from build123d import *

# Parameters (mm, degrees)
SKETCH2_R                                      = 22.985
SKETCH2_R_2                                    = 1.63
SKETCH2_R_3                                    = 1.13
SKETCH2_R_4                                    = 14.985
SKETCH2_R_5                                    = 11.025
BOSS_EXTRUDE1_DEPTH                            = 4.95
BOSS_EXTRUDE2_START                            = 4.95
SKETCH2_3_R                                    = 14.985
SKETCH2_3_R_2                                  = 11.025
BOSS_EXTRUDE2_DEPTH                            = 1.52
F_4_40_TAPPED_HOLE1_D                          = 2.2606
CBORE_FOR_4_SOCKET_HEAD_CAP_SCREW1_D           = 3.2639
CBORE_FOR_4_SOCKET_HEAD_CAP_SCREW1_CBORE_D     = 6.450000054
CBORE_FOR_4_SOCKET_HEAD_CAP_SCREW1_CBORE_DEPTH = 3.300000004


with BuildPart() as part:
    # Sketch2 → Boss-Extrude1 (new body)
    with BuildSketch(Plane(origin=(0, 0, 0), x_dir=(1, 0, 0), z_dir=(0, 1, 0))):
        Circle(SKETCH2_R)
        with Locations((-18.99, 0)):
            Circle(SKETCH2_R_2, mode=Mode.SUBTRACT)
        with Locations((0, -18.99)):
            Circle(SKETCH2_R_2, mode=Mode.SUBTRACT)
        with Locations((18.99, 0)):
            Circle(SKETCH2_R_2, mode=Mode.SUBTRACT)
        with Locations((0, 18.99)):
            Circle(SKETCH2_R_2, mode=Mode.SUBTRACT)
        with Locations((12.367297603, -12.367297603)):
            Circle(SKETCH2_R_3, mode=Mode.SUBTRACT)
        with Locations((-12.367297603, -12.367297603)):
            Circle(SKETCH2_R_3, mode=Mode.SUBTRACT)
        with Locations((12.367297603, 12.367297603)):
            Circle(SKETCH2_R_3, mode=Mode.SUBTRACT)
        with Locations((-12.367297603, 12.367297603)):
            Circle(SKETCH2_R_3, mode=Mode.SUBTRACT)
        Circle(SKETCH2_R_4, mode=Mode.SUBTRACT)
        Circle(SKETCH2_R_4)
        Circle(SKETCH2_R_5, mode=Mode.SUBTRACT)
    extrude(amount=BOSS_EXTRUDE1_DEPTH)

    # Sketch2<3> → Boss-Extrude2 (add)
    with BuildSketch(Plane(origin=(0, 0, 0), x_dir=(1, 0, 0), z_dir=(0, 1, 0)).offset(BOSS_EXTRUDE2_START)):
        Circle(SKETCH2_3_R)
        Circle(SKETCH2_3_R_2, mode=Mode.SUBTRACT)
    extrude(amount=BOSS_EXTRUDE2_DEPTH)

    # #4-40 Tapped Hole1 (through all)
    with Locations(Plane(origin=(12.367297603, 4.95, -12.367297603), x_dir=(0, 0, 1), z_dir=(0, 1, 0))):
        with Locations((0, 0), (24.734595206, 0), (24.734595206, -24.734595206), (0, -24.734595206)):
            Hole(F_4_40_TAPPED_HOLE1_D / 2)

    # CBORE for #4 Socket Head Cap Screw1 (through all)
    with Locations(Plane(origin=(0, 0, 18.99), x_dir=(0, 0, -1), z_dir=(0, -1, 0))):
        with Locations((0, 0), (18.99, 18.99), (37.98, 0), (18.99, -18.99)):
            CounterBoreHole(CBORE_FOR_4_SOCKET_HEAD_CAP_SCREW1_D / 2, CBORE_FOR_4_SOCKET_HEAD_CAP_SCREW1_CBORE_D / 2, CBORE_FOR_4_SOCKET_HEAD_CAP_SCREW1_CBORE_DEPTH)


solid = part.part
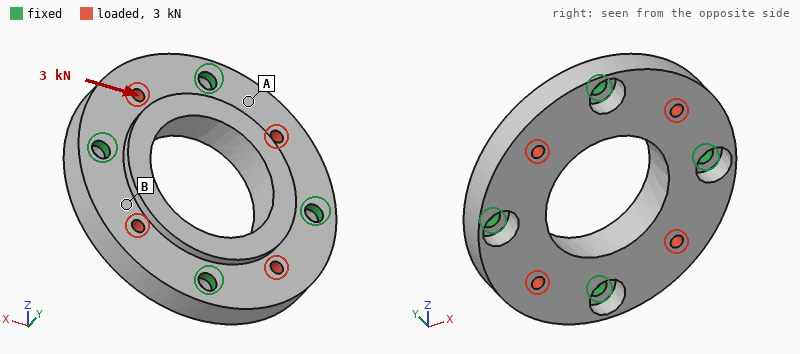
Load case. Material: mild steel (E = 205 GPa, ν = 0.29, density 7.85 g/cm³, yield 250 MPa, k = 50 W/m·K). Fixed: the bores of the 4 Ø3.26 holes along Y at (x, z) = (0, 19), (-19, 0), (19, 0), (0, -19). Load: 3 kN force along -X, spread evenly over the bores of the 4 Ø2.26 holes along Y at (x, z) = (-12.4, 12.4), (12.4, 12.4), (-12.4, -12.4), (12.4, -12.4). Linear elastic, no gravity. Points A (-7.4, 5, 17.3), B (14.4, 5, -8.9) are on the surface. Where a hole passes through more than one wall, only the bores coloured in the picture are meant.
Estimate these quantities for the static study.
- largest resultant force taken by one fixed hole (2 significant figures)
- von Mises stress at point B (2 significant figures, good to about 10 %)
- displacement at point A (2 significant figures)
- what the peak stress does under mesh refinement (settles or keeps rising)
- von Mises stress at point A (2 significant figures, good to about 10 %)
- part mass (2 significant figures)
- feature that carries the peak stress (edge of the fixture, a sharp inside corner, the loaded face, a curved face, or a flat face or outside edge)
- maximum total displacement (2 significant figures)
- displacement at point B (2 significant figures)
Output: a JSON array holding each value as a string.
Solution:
["910 N", "11 MPa", "1.3 µm", "keeps rising", "23 MPa", "49 g", "edge of the fixture", "2.6 µm", "1.4 µm"]
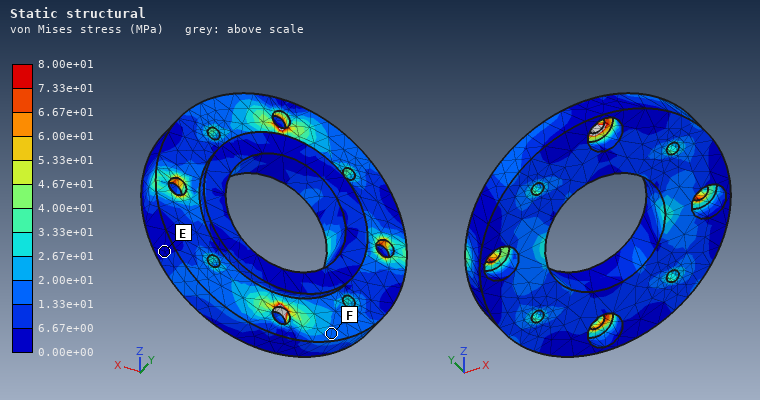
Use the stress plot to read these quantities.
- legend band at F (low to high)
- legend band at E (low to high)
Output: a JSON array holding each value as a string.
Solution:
["1.33e+01 to 2.00e+01 MPa", "0.00e+00 to 6.67e+00 MPa"]
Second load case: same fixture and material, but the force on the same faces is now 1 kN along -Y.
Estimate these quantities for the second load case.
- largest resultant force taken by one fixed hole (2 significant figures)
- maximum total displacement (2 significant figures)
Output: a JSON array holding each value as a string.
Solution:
["260 N", "2.7 µm"]
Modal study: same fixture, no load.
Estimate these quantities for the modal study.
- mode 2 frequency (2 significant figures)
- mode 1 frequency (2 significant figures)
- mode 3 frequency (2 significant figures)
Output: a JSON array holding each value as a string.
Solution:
["18 kHz", "15 kHz", "18 kHz"]
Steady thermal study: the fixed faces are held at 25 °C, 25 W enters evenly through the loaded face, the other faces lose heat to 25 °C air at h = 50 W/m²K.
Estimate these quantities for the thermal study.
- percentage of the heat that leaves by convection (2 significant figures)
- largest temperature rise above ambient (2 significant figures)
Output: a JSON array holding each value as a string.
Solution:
["12 %", "25 K"]
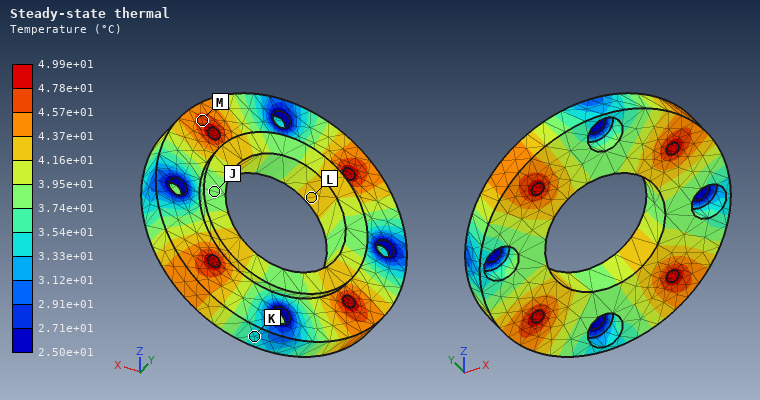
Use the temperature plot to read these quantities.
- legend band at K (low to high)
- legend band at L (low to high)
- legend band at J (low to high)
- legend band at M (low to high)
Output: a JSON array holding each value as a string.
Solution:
["3.33e+01 to 3.54e+01 °C", "4.16e+01 to 4.37e+01 °C", "3.74e+01 to 3.95e+01 °C", "4.57e+01 to 4.78e+01 °C"]
